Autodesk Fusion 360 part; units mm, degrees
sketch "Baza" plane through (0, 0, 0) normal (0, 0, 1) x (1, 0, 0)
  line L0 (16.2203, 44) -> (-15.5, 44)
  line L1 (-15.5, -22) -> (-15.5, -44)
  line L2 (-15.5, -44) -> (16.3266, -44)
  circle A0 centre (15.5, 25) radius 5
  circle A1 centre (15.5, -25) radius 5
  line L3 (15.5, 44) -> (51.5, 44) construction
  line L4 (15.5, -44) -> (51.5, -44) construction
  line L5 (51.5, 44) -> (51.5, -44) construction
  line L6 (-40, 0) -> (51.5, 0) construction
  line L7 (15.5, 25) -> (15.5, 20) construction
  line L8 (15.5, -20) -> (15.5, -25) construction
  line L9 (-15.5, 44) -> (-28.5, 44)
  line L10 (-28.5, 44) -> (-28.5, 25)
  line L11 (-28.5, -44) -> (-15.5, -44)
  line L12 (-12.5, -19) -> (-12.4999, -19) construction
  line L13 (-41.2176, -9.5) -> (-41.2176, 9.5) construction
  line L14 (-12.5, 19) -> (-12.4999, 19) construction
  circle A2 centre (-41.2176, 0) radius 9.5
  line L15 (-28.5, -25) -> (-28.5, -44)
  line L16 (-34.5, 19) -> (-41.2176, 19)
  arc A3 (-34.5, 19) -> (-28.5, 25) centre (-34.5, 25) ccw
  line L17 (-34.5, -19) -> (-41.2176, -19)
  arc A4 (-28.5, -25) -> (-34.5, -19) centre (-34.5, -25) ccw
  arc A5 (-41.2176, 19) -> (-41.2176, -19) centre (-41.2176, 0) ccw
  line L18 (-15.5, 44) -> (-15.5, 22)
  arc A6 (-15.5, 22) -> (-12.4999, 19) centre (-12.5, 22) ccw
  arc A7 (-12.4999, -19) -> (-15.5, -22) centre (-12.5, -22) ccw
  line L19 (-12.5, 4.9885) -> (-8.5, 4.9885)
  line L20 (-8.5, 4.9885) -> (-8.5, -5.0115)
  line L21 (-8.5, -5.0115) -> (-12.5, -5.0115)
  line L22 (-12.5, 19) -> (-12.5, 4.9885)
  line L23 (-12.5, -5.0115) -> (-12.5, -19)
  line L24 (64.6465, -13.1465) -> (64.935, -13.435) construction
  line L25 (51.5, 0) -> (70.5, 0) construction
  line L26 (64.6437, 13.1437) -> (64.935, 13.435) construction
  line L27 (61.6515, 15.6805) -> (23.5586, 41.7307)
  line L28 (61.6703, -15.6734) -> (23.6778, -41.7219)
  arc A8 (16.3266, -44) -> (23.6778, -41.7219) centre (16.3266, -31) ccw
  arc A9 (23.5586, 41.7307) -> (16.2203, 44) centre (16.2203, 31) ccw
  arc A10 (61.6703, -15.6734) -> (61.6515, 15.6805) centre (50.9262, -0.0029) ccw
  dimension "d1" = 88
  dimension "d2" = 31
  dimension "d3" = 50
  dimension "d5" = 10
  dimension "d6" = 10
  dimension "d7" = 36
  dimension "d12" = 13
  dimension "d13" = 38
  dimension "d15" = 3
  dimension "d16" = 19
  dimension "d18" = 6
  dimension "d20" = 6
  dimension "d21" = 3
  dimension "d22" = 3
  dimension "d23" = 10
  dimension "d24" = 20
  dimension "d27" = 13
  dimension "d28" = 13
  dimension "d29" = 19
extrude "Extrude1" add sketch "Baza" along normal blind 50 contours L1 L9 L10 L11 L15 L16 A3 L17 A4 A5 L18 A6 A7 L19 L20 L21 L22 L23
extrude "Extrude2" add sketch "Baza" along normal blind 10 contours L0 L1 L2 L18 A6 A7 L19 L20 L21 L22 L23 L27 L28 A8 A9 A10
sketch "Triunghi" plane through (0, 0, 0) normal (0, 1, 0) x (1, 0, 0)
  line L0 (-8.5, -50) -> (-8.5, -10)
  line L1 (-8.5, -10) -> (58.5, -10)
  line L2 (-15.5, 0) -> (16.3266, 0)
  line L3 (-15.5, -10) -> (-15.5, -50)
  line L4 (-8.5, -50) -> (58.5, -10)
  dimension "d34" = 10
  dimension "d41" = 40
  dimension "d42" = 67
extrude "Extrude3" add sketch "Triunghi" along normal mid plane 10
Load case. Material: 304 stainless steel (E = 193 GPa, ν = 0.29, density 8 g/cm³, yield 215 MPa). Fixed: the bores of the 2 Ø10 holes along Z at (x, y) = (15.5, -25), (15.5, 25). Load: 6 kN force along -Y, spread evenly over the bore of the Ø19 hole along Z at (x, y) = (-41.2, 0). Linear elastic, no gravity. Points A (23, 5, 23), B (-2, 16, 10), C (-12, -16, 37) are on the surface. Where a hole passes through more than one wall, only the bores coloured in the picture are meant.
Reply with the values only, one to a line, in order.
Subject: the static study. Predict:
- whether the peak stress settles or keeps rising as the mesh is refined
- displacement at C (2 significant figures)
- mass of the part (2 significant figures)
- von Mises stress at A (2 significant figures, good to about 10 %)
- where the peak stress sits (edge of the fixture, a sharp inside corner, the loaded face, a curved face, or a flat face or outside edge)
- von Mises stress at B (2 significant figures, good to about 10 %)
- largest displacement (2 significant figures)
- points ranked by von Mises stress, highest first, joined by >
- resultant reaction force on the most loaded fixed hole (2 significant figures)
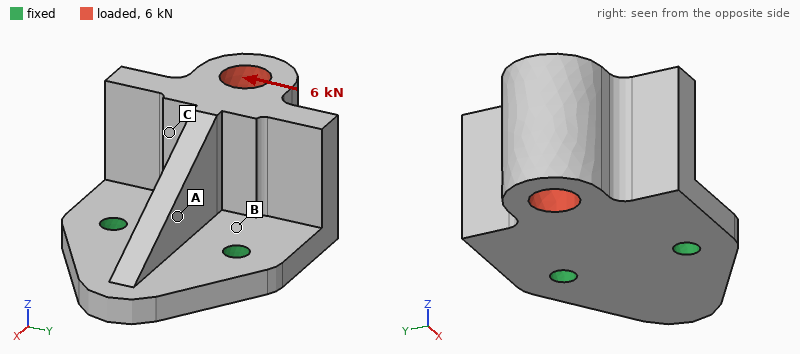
keeps rising
18 µm
1.4 kg
14 MPa
edge of the fixture
37 MPa
32 µm
B > A > C
7.1 kN
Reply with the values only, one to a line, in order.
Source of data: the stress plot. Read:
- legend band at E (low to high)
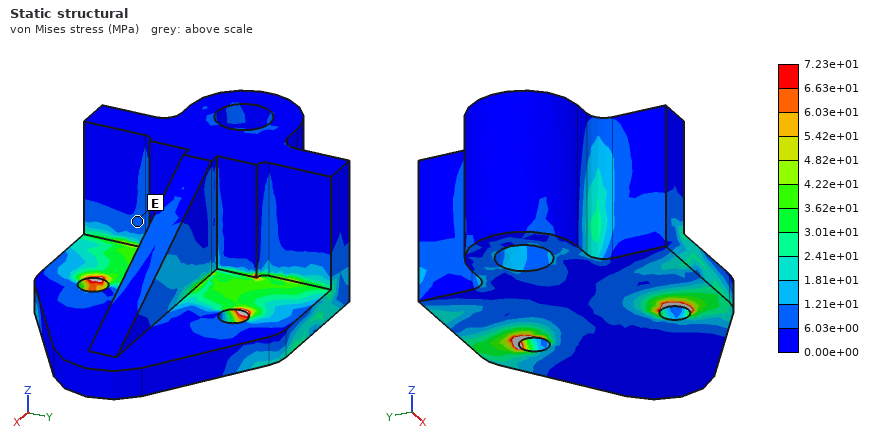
6.03e+00 to 1.21e+01 MPa
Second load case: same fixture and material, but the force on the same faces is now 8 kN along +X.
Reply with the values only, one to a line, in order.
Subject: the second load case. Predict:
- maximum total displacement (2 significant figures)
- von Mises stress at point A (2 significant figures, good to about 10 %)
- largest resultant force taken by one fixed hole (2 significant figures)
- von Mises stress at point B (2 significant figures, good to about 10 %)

85 µm
21 MPa
4.0 kN
27 MPa
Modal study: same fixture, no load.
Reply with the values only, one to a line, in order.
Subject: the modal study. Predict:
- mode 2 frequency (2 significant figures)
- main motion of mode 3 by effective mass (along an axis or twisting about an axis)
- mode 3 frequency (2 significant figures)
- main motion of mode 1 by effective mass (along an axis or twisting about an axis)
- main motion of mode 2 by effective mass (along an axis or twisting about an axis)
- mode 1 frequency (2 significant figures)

2600 Hz
along Z
5300 Hz
along Z
along Y
1400 Hz
